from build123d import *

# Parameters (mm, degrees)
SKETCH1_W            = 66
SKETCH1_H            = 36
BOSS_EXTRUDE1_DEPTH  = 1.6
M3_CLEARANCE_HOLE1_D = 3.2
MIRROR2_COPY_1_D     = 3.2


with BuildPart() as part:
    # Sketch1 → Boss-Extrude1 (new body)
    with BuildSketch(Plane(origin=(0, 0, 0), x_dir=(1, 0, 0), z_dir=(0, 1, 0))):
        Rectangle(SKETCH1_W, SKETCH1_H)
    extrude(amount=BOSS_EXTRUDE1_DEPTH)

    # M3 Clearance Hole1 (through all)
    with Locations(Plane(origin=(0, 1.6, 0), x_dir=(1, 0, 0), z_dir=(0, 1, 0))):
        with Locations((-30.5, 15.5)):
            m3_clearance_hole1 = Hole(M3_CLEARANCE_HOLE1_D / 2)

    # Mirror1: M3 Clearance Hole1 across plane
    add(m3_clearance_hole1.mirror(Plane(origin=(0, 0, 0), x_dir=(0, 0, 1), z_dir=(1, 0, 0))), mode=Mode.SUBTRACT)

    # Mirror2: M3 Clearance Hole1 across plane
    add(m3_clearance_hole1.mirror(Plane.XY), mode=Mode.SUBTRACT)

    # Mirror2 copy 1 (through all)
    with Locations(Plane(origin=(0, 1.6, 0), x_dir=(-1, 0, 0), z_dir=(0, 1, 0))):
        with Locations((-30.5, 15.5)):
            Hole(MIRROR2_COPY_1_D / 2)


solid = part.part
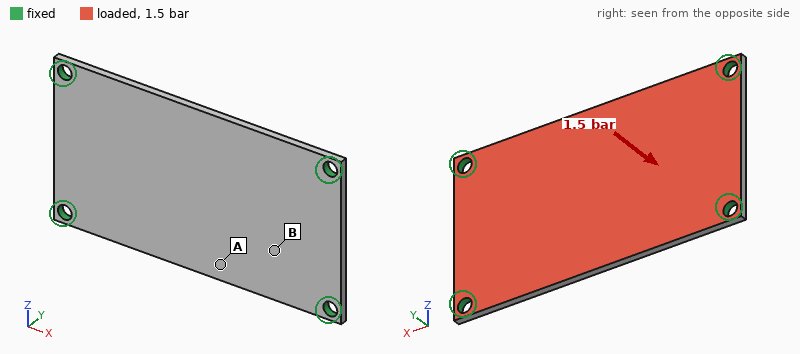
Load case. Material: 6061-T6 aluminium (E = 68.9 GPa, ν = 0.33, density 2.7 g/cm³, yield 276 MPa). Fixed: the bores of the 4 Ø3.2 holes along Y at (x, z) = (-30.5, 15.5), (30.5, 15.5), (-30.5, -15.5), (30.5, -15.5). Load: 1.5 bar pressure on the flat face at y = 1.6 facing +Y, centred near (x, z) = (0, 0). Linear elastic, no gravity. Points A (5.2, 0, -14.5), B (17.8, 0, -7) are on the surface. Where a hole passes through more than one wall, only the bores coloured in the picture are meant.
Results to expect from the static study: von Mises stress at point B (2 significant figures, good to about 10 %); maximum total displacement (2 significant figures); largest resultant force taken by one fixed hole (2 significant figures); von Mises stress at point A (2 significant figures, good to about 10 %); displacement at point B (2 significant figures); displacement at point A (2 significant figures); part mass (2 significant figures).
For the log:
18 MPa
0.28 mm
88 N
58 MPa
0.14 mm
0.26 mm
10 g
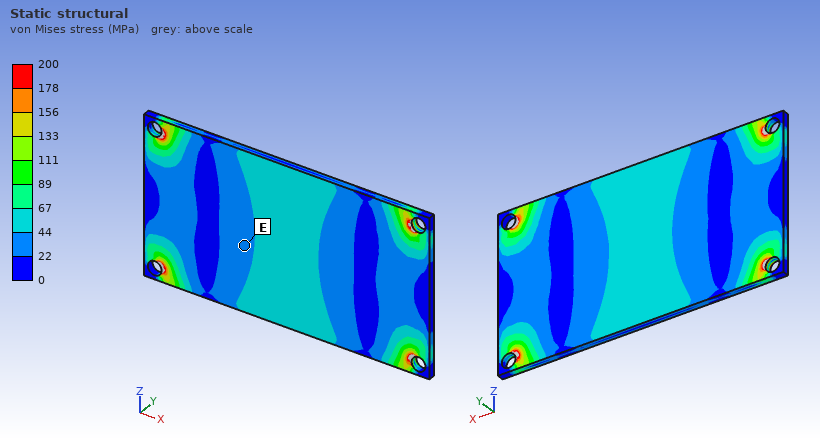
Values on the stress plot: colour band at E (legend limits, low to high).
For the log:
22 to 44 MPa
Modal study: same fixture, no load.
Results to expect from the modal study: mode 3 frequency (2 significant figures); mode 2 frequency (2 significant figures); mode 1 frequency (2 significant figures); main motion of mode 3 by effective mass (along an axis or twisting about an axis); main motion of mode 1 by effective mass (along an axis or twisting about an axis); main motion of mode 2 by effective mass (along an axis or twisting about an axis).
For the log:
5500 Hz
3500 Hz
2000 Hz
twisting about Z
along Y
twisting about X
